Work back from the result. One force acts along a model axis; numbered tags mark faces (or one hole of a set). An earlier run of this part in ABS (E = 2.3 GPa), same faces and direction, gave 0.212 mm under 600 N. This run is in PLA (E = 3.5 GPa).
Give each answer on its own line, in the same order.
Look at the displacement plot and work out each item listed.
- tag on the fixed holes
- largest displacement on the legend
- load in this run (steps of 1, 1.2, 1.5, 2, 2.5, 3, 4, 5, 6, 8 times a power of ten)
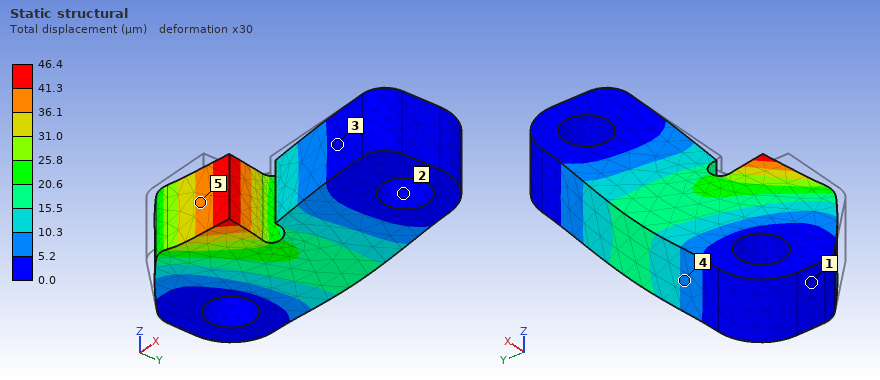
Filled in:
2
46.4 µm
200 N
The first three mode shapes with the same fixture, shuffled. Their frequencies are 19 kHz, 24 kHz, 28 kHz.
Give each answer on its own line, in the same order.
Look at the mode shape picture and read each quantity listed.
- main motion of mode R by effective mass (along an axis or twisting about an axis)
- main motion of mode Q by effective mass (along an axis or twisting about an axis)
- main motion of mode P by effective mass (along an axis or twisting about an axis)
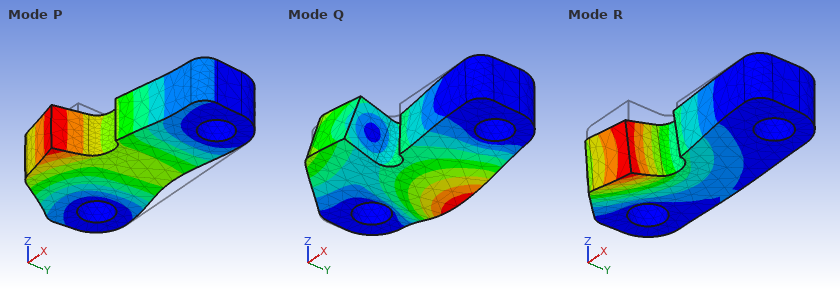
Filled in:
along Z
along Z
along Y
